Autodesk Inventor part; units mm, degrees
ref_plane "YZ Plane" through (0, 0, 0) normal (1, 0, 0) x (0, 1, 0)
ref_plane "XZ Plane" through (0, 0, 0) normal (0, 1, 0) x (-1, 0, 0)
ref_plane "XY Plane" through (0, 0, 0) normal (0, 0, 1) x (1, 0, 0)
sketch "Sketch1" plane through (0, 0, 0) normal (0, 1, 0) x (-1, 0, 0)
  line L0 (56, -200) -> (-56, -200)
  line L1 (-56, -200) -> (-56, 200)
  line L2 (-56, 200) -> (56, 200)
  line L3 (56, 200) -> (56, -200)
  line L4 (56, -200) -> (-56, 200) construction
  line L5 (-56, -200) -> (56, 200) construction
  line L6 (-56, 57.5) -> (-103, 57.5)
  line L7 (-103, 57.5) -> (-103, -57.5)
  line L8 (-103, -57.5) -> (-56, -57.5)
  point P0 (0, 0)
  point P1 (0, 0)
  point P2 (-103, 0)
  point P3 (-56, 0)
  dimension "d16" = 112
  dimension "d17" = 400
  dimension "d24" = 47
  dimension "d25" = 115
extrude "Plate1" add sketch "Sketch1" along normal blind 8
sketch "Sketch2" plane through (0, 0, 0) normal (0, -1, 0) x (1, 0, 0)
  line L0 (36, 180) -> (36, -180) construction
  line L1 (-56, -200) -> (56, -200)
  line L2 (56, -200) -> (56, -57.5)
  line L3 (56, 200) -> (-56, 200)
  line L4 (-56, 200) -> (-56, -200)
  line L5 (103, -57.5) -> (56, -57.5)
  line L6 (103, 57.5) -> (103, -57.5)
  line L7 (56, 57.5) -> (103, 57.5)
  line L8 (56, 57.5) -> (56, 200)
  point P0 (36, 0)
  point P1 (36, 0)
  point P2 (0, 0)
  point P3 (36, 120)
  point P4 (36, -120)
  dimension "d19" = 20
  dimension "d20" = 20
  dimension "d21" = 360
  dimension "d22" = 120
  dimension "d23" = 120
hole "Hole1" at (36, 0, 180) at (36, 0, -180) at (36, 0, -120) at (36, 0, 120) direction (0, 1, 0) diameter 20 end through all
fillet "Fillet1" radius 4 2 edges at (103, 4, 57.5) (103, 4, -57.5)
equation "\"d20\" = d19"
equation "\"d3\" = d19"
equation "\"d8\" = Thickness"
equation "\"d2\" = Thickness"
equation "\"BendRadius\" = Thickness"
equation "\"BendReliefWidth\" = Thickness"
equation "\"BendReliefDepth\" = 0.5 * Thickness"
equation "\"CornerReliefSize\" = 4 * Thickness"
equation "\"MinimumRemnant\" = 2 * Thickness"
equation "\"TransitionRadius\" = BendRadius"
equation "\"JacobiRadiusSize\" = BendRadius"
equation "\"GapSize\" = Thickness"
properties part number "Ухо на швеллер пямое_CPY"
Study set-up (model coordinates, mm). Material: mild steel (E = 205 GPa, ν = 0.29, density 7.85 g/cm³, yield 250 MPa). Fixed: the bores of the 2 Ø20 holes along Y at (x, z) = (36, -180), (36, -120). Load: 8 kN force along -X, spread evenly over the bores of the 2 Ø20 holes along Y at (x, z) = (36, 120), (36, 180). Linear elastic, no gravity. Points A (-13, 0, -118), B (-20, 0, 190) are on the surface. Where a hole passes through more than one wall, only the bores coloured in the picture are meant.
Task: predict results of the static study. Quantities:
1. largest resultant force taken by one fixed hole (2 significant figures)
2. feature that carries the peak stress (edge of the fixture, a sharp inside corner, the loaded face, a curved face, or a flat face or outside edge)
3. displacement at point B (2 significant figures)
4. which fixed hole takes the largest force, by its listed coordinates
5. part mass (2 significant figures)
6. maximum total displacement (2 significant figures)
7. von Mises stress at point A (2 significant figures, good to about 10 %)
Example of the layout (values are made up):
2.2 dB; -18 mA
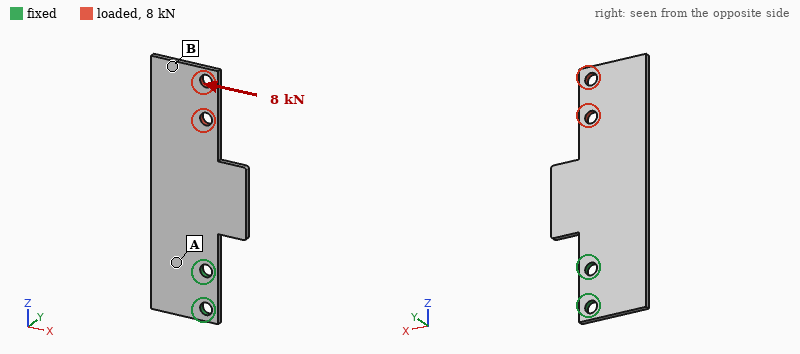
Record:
35 kN; edge of the fixture; 0.57 mm; (36, -120); 3.1 kg; 0.61 mm; 67 MPa
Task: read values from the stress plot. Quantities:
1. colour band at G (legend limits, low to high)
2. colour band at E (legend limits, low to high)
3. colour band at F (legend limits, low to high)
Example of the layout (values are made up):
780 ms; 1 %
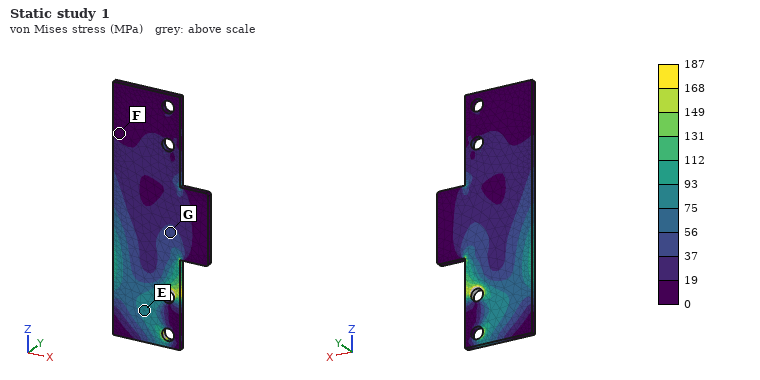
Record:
37 to 56 MPa; 75 to 93 MPa; 0 to 19 MPa
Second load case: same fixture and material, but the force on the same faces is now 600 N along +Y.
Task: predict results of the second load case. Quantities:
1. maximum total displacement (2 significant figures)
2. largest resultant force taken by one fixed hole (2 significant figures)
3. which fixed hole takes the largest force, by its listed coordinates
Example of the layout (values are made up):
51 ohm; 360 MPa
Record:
5.0 mm; 1.4 kN; (36, -120)
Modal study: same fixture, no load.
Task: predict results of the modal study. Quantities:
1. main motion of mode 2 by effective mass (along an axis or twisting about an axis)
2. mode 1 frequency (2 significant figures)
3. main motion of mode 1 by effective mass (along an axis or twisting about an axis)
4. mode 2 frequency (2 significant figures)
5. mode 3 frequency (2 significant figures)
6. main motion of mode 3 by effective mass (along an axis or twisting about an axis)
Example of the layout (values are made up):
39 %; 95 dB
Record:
twisting about Z; 66 Hz; along Y; 290 Hz; 370 Hz; along Y
